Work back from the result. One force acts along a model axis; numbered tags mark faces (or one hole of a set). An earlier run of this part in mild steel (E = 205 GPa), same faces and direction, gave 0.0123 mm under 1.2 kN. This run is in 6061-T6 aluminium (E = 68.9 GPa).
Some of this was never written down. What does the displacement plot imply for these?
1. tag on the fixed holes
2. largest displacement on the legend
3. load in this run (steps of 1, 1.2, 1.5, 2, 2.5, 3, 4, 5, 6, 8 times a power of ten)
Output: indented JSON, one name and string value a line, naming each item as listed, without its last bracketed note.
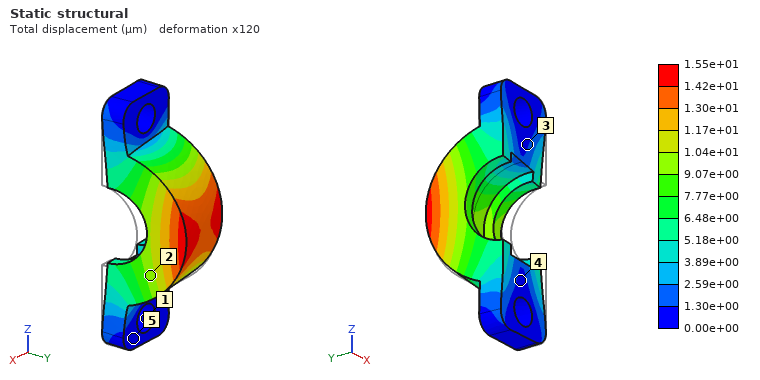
{
  "tag on the fixed holes": "1",
  "largest displacement on the legend": "1.55e+01 µm",
  "load in this run": "500 N"
}
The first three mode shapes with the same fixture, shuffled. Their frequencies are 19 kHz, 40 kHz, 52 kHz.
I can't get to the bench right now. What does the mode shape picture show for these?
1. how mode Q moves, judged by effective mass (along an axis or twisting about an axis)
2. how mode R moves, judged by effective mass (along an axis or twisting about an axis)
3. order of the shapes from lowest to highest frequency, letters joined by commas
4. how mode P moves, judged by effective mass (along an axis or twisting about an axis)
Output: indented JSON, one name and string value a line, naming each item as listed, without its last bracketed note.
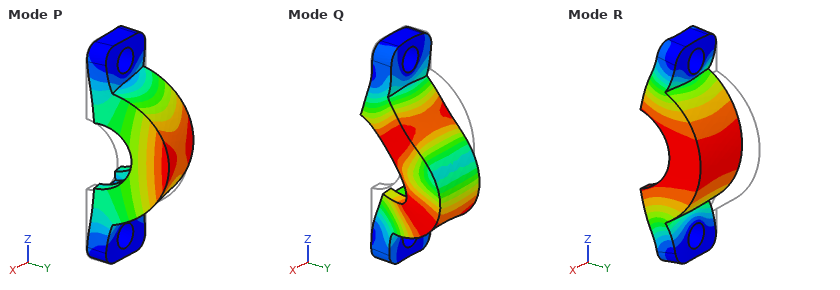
{
  "how mode Q moves, judged by effective mass": "along Z",
  "how mode R moves, judged by effective mass": "along Y",
  "order of the shapes from lowest to highest frequency, letters joined by commas": "P, R, Q",
  "how mode P moves, judged by effective mass": "along X"
}
